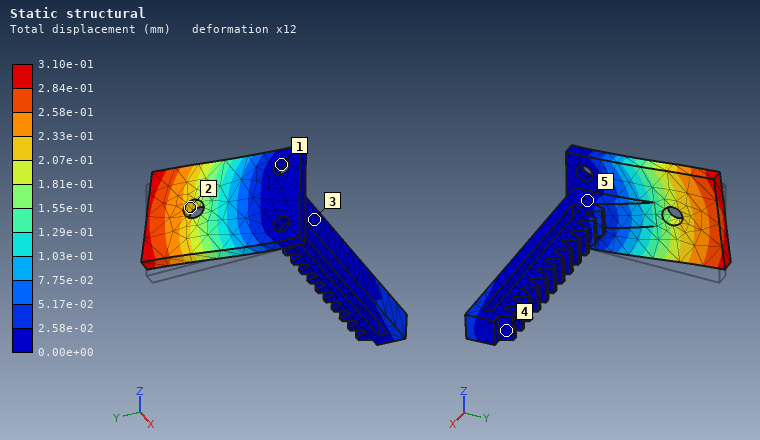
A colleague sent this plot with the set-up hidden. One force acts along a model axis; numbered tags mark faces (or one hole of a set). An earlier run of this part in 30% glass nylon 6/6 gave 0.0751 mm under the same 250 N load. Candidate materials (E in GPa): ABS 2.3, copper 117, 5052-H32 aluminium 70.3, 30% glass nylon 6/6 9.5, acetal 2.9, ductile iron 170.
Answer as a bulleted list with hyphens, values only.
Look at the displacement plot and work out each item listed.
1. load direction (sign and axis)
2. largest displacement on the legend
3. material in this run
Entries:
- +Z
- 3.10e-01 mm
- ABS
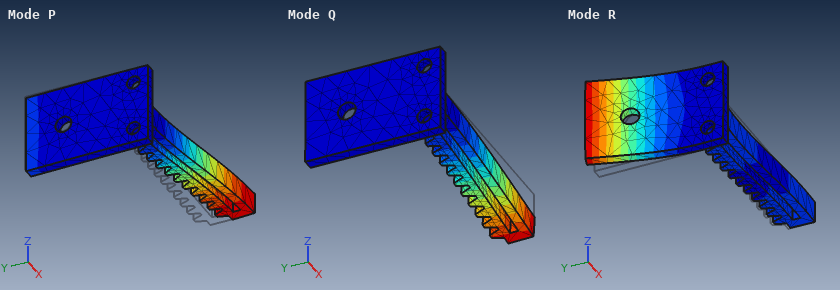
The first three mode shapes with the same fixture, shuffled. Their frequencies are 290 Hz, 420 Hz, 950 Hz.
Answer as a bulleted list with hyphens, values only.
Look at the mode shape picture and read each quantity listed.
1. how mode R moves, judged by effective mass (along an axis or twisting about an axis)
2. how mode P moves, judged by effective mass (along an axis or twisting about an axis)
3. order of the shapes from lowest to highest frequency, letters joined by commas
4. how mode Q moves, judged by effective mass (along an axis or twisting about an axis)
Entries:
- along X
- along Y
- P, Q, R
- along Z
